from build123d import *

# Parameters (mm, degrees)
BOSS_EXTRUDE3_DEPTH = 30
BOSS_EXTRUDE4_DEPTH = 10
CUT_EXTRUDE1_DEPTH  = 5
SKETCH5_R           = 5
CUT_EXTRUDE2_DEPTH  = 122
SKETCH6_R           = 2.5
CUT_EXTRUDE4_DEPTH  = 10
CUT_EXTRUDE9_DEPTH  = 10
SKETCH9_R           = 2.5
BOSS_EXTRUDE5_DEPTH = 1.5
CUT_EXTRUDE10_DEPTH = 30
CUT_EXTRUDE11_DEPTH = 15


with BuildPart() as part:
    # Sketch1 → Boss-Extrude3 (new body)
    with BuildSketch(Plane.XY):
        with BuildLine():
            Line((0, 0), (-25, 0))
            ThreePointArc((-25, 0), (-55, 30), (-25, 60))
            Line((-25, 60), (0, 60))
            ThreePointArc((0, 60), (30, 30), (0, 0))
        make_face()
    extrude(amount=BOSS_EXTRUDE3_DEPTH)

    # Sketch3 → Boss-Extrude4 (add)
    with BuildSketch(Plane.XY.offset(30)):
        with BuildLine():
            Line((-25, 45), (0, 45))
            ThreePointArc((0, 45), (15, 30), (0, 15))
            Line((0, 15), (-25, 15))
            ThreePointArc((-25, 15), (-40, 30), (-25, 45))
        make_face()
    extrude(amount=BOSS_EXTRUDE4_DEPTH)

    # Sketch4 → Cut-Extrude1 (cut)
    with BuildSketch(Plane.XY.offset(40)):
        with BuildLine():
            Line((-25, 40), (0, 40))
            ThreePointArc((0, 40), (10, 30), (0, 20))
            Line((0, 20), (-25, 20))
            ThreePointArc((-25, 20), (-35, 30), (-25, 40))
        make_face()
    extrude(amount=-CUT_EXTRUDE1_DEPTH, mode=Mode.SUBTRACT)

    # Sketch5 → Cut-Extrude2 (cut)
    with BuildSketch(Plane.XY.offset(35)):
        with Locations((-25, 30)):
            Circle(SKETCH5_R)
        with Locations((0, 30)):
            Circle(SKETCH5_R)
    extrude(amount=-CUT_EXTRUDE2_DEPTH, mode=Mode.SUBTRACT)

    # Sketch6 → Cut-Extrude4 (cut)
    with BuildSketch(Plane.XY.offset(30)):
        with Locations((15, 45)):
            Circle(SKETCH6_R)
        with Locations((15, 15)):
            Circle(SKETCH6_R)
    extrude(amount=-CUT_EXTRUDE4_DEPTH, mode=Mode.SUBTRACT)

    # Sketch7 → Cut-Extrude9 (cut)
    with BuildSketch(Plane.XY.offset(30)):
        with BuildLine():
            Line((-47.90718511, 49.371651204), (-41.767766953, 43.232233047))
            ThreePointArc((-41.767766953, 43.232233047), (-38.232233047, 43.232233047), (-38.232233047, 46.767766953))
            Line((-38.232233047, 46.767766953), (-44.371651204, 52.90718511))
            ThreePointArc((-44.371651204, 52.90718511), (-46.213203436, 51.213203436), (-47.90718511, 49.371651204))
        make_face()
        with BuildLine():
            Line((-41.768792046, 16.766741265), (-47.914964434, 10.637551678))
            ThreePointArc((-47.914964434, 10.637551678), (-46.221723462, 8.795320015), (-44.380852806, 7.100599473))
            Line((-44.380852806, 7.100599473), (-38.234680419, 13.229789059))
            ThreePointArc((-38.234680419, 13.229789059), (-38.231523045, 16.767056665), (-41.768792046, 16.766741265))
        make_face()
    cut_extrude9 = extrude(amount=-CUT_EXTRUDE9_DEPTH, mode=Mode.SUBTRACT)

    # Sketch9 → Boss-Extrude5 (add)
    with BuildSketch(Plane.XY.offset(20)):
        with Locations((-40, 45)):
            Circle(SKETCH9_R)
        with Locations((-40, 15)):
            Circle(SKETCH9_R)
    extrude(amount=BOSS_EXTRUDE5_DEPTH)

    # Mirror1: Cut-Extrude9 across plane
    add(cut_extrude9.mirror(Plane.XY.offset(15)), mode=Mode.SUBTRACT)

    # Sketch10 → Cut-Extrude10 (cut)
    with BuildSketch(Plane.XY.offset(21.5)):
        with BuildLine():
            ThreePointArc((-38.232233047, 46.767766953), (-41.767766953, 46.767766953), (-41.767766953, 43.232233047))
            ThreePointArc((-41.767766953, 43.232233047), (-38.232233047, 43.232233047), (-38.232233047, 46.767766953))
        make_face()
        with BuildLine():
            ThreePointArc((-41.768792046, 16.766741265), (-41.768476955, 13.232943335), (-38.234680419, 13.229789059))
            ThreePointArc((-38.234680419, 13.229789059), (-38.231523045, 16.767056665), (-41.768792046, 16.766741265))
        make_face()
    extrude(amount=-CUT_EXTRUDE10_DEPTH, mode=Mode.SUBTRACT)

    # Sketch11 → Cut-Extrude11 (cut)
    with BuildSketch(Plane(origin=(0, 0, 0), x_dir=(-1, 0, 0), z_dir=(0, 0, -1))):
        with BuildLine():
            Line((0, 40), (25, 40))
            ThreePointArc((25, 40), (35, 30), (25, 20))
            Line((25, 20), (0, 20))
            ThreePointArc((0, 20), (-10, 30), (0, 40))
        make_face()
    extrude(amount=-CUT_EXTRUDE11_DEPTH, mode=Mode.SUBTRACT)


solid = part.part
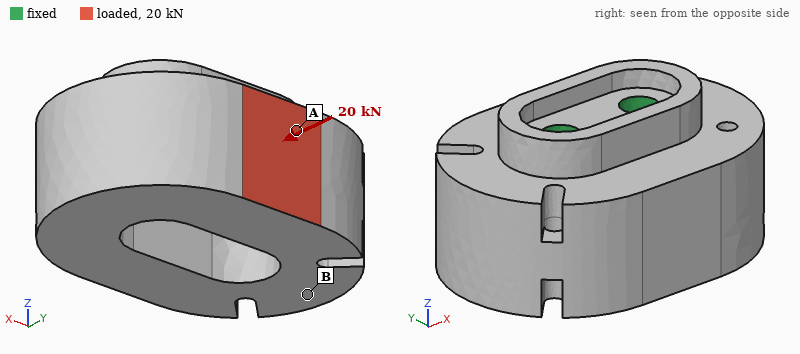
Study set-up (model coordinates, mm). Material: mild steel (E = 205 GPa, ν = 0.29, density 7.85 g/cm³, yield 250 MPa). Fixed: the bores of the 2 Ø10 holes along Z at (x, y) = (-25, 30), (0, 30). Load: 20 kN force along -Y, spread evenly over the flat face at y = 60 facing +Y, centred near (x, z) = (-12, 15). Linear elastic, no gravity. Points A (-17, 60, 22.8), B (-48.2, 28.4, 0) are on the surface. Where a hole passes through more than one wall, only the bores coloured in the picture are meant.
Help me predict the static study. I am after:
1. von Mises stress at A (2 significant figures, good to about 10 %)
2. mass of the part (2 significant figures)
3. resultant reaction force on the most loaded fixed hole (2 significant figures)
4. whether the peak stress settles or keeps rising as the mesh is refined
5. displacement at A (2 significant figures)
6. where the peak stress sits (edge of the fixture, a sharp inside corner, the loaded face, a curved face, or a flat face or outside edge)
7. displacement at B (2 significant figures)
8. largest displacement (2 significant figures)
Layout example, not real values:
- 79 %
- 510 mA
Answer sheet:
- 25 MPa
- 960 g
- 11 kN
- keeps rising
- 7.4 µm
- edge of the fixture
- 5.0 µm
- 15 µm
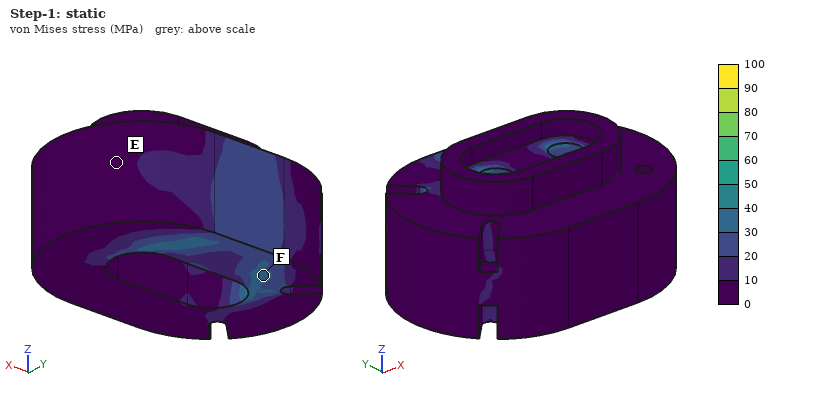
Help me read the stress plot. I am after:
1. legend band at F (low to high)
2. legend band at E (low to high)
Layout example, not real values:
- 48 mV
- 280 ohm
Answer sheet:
- 30 to 40 MPa
- 0 to 10 MPa
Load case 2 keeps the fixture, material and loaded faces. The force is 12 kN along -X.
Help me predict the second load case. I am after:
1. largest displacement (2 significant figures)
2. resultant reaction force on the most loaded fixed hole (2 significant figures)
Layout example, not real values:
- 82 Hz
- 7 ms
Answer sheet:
- 7.5 µm
- 12 kN
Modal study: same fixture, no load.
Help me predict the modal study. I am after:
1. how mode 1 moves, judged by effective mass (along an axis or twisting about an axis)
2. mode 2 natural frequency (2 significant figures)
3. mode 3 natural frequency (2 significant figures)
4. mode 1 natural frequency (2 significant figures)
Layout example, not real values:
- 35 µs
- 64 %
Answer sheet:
- along Y
- 11 kHz
- 11 kHz
- 9000 Hz
